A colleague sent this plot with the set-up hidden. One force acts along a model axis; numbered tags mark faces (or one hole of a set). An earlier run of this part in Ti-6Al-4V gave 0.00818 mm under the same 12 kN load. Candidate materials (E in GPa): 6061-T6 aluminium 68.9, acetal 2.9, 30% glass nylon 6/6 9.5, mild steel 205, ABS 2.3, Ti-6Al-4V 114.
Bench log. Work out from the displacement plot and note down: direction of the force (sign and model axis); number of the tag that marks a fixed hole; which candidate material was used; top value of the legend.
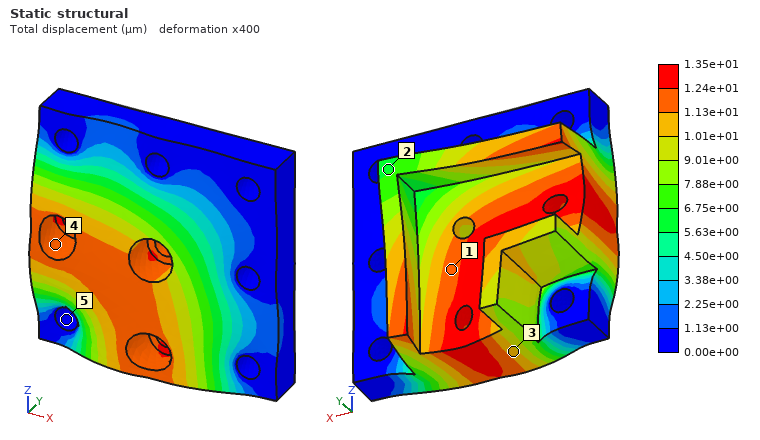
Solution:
-Y
5
6061-T6 aluminium
1.35e+01 µm
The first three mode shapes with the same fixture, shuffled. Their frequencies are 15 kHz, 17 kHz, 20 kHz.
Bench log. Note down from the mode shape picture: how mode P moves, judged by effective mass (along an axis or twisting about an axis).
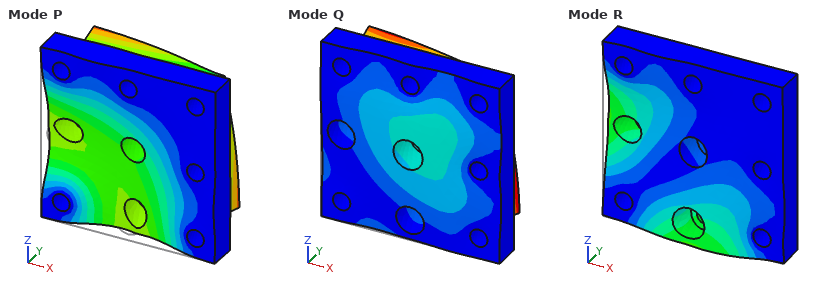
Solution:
along Y
